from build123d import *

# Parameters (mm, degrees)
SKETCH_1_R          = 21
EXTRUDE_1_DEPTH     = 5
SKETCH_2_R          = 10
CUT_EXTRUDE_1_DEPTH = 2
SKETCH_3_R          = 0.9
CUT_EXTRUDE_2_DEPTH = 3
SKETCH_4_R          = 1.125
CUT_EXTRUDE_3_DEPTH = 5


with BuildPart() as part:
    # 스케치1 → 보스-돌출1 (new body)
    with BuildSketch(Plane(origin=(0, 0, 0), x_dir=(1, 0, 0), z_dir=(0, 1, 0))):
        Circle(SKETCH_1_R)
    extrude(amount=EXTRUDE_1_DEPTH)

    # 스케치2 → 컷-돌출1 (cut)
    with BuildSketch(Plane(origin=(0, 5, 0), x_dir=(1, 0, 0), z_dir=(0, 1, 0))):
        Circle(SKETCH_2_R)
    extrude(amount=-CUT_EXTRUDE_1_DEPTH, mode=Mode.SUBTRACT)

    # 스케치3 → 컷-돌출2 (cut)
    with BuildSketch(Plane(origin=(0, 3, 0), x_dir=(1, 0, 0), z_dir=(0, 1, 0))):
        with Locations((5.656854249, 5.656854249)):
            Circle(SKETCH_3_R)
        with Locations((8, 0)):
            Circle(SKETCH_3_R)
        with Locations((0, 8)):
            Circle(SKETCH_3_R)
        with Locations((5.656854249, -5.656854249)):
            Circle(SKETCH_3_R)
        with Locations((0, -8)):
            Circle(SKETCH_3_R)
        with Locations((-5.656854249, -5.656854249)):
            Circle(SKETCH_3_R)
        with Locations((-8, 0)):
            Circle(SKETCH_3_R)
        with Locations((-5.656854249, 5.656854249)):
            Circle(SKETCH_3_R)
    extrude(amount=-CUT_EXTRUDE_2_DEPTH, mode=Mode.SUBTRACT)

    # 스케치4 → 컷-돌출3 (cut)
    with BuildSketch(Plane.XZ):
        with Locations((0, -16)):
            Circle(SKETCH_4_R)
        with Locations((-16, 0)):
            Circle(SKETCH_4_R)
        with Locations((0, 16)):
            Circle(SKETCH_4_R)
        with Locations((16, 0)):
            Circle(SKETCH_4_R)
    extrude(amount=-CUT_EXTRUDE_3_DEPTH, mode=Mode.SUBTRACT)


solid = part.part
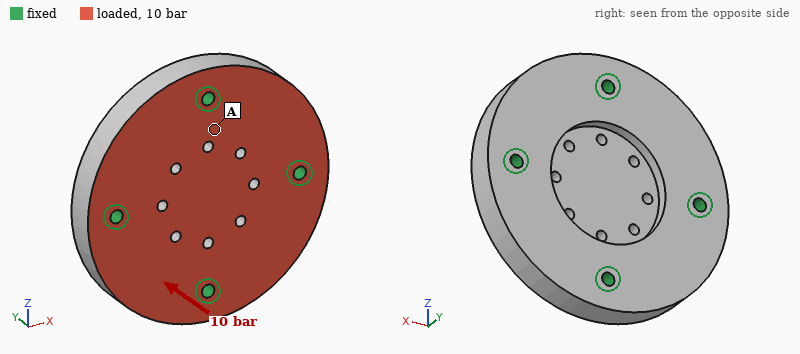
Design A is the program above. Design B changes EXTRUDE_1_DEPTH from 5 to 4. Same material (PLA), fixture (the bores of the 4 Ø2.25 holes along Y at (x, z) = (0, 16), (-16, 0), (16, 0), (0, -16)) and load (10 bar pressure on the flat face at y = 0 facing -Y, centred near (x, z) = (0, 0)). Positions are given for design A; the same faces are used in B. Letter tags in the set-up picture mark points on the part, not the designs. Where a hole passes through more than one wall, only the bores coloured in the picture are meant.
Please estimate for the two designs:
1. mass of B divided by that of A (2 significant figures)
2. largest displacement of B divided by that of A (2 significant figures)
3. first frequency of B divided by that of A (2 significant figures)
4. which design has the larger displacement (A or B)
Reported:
0.83
1.4
0.87
B
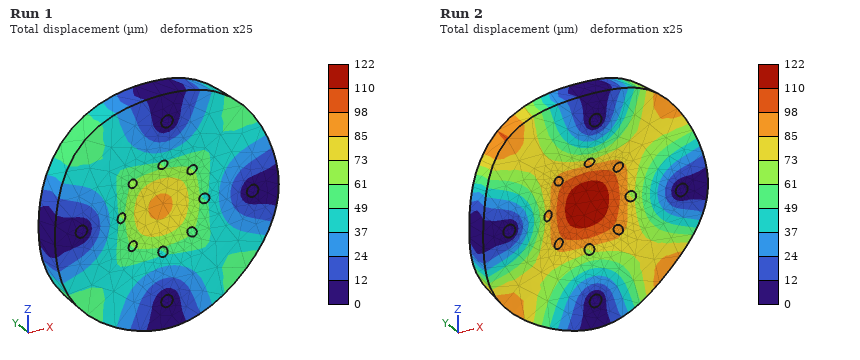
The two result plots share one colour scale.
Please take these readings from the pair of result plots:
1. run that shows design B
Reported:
Run 2
